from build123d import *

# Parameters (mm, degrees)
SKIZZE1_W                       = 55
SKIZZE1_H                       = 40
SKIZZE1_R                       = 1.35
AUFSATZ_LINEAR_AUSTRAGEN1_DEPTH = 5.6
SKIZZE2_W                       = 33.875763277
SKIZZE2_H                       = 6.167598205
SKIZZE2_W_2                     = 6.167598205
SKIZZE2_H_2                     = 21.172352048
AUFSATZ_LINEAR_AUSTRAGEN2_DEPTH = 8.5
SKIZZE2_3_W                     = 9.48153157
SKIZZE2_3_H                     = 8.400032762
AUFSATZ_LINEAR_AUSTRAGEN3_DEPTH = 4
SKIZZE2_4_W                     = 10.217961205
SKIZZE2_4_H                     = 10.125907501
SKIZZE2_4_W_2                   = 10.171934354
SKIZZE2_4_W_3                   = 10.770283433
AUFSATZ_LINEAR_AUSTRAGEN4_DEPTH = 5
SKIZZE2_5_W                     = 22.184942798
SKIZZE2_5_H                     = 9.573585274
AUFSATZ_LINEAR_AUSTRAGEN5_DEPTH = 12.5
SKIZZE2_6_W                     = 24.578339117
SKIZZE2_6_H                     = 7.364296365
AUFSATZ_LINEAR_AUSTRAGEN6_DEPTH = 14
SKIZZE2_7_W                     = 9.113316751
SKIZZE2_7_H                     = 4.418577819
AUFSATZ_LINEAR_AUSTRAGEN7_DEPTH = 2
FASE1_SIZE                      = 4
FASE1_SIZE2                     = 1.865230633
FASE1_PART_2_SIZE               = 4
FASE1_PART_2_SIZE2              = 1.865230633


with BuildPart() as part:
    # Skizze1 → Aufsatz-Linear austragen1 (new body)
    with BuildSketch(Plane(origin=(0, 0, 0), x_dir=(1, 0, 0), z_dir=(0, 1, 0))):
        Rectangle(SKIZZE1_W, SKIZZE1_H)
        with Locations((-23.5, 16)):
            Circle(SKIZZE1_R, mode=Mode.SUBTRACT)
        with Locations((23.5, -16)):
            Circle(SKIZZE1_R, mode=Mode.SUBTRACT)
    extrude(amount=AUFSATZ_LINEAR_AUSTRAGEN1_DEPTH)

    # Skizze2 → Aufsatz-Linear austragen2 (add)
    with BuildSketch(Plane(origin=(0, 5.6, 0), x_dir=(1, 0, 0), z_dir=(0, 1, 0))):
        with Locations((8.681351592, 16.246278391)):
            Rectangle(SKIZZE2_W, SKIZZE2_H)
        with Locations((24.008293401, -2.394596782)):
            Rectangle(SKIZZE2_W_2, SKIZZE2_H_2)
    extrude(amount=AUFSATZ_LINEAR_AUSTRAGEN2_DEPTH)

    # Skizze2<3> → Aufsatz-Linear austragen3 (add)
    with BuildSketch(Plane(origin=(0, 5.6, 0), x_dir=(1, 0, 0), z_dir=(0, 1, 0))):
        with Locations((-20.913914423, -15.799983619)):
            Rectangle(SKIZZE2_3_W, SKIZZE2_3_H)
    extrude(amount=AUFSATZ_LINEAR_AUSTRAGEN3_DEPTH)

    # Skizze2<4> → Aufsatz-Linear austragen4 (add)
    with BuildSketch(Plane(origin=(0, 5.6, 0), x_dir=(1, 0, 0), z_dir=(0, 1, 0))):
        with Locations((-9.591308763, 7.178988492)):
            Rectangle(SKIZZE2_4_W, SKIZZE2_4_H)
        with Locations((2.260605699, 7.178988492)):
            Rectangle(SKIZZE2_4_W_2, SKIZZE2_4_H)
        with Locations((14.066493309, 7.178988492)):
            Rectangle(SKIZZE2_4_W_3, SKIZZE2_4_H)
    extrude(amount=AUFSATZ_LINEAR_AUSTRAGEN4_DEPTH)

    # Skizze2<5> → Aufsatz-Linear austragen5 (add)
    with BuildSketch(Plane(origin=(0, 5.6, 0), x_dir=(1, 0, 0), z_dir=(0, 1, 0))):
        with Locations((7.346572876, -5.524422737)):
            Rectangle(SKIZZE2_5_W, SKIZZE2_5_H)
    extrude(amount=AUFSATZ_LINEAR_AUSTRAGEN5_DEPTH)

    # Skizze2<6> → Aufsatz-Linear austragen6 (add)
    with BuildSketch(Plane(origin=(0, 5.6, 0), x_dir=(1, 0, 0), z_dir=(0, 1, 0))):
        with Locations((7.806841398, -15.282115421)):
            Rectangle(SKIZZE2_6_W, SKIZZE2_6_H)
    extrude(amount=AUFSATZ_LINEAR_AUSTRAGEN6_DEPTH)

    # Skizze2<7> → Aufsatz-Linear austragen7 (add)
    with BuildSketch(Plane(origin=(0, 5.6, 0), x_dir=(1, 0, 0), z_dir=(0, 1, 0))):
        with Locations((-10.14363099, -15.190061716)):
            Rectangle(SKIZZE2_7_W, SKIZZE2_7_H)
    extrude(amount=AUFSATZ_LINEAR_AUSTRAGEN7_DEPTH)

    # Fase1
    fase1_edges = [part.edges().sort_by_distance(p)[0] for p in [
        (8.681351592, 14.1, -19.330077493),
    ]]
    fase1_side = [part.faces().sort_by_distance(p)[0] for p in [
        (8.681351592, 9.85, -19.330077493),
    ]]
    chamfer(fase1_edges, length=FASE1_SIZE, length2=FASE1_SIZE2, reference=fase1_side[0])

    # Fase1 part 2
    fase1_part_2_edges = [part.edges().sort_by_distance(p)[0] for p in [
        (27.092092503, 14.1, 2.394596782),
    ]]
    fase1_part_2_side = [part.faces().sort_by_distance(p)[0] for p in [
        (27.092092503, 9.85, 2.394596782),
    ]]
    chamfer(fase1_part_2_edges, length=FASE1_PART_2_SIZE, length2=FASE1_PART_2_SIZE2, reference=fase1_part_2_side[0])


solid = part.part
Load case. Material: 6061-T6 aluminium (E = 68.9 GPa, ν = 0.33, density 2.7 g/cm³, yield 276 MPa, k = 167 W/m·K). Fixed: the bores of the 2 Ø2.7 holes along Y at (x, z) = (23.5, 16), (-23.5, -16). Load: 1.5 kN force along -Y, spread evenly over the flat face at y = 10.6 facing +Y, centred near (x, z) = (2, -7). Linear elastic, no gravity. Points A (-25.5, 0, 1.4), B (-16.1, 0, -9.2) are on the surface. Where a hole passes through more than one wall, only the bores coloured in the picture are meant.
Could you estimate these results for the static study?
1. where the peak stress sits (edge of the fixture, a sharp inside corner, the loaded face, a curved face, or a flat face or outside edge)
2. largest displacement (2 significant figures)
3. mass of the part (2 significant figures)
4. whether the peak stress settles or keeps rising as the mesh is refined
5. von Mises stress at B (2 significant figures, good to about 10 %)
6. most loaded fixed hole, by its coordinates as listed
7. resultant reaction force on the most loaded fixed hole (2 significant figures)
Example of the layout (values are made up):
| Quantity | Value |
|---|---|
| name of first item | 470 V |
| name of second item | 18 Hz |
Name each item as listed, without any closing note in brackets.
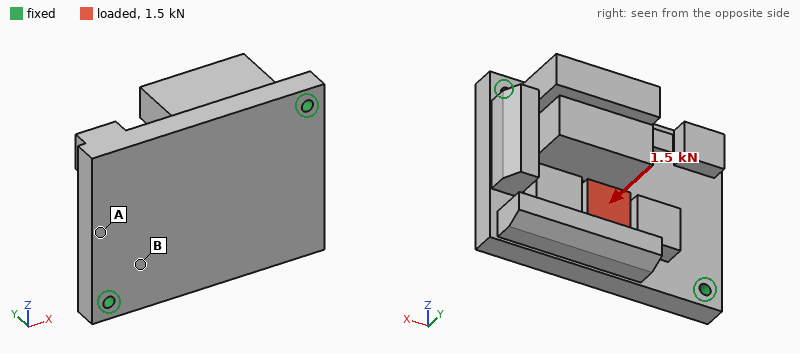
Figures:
| Quantity | Value |
|---|---|
| where the peak stress sits | edge of the fixture |
| largest displacement | 0.13 mm |
| mass of the part | 60 g |
| whether the peak stress settles or keeps rising as the mesh is refined | keeps rising |
| von Mises stress at B | 29 MPa |
| most loaded fixed hole, by its coordinates as listed | (-23.5, -16) |
| resultant reaction force on the most loaded fixed hole | 870 N |
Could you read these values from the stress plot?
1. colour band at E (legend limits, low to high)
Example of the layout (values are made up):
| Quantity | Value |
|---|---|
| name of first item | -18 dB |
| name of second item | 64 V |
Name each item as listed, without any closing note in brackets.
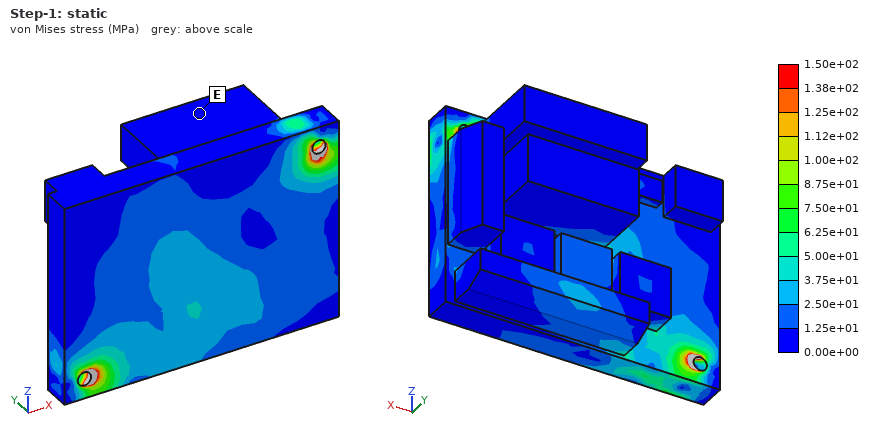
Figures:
| Quantity | Value |
|---|---|
| colour band at E | 0.00e+00 to 1.25e+01 MPa |
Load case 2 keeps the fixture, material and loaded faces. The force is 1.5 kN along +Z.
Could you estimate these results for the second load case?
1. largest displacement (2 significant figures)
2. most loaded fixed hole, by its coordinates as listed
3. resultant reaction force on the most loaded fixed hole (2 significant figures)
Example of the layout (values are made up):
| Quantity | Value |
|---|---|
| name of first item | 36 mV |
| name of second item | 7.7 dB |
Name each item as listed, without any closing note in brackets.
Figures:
| Quantity | Value |
|---|---|
| largest displacement | 85 µm |
| most loaded fixed hole, by its coordinates as listed | (23.5, 16) |
| resultant reaction force on the most loaded fixed hole | 830 N |
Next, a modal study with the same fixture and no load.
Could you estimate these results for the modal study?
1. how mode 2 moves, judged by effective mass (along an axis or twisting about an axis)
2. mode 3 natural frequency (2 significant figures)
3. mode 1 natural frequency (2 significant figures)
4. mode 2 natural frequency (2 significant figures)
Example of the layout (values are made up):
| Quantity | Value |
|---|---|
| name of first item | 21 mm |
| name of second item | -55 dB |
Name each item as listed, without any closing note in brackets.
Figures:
| Quantity | Value |
|---|---|
| how mode 2 moves, judged by effective mass | along Y |
| mode 3 natural frequency | 10 kHz |
| mode 1 natural frequency | 2900 Hz |
| mode 2 natural frequency | 4500 Hz |
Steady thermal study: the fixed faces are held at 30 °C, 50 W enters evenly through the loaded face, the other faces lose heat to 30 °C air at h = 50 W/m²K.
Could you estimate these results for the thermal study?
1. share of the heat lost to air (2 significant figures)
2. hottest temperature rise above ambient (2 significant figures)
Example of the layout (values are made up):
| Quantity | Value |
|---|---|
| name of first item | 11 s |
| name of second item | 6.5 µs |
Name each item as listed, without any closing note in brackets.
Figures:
| Quantity | Value |
|---|---|
| share of the heat lost to air | 15 % |
| hottest temperature rise above ambient | 46 K |
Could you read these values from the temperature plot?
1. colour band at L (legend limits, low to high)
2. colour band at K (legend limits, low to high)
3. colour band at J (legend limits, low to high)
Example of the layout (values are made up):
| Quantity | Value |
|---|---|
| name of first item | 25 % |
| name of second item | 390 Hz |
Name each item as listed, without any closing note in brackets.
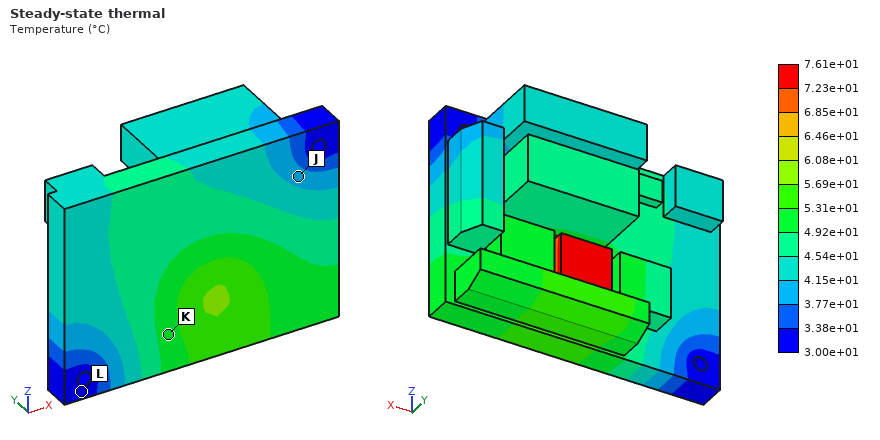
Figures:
| Quantity | Value |
|---|---|
| colour band at L | 3.00e+01 to 3.38e+01 °C |
| colour band at K | 4.92e+01 to 5.31e+01 °C |
| colour band at J | 3.77e+01 to 4.15e+01 °C |
